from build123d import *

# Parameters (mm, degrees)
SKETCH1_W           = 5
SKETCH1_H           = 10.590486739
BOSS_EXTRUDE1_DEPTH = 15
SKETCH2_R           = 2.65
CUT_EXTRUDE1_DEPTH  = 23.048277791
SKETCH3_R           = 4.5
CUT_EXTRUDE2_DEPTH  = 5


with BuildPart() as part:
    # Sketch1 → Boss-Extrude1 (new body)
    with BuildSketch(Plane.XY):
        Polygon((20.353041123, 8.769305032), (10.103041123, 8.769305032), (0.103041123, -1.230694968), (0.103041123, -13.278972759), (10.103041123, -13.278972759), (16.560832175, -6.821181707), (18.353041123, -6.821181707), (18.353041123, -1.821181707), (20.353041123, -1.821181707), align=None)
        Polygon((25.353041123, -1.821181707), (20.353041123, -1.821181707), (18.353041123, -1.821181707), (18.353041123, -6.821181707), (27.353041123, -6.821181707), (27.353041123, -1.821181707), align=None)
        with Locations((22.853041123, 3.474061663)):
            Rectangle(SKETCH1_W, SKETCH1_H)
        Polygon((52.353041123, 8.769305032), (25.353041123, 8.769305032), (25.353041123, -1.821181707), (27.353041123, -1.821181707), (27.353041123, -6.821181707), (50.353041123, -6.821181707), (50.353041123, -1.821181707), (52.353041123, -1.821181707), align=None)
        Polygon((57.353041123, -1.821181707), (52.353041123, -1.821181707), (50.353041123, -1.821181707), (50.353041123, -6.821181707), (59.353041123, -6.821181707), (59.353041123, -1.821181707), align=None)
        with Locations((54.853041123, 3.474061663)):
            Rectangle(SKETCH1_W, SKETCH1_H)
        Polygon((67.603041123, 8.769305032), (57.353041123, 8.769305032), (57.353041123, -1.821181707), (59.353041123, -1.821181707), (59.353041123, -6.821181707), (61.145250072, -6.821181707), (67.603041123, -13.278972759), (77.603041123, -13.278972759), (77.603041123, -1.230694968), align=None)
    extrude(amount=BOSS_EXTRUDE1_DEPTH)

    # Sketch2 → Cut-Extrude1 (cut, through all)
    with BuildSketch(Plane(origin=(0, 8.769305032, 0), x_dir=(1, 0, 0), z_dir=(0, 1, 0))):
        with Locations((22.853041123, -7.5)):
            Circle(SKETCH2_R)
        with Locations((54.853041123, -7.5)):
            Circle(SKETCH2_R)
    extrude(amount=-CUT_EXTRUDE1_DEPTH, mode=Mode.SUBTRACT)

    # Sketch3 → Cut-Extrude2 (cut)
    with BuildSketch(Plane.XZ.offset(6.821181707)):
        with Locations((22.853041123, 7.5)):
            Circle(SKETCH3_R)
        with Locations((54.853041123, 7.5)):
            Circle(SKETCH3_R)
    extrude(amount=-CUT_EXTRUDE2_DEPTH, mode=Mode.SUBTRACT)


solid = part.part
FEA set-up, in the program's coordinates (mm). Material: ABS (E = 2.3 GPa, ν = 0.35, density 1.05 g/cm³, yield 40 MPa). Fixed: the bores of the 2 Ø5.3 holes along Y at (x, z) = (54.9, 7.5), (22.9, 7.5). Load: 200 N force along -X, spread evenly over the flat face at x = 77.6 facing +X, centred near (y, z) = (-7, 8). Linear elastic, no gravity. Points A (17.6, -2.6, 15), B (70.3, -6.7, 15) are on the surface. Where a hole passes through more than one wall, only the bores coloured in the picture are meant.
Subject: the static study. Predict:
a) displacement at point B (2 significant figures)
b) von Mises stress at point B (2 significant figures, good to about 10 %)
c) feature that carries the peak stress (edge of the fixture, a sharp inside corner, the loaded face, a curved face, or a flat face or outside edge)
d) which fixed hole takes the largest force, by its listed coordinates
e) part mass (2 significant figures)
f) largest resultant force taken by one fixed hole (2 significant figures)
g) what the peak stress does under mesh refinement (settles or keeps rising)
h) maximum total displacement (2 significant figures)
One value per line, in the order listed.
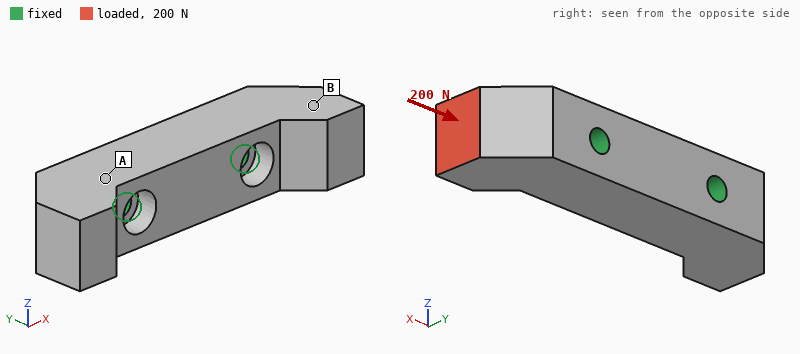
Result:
52 µm
1.8 MPa
edge of the fixture
(54.9, 7.5)
19 g
160 N
keeps rising
91 µm
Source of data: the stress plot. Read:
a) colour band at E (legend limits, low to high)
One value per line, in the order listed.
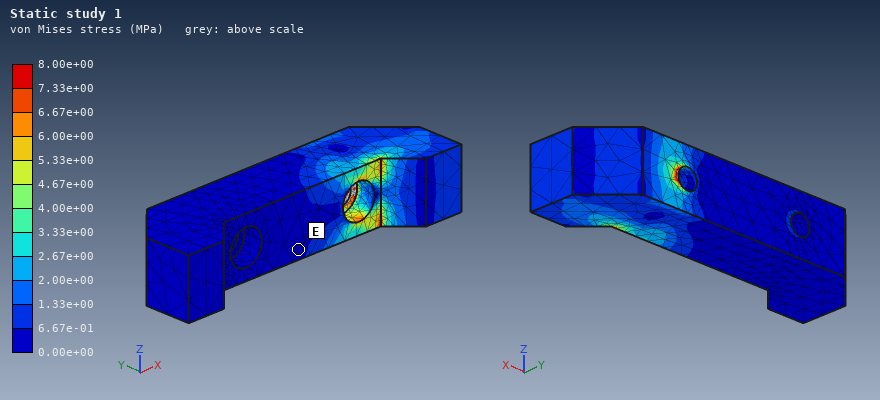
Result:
0.00e+00 to 6.67e-01 MPa
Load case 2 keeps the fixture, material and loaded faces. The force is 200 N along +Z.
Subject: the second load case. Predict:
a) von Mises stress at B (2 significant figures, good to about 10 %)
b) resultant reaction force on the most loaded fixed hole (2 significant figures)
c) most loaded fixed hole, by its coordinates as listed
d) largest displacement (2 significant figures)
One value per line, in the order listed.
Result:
3.1 MPa
270 N
(54.9, 7.5)
0.24 mm
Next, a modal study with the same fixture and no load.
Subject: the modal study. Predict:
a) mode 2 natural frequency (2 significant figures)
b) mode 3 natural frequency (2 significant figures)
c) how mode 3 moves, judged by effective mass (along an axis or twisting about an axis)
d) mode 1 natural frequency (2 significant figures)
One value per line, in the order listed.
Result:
3700 Hz
3900 Hz
along Y
3600 Hz
